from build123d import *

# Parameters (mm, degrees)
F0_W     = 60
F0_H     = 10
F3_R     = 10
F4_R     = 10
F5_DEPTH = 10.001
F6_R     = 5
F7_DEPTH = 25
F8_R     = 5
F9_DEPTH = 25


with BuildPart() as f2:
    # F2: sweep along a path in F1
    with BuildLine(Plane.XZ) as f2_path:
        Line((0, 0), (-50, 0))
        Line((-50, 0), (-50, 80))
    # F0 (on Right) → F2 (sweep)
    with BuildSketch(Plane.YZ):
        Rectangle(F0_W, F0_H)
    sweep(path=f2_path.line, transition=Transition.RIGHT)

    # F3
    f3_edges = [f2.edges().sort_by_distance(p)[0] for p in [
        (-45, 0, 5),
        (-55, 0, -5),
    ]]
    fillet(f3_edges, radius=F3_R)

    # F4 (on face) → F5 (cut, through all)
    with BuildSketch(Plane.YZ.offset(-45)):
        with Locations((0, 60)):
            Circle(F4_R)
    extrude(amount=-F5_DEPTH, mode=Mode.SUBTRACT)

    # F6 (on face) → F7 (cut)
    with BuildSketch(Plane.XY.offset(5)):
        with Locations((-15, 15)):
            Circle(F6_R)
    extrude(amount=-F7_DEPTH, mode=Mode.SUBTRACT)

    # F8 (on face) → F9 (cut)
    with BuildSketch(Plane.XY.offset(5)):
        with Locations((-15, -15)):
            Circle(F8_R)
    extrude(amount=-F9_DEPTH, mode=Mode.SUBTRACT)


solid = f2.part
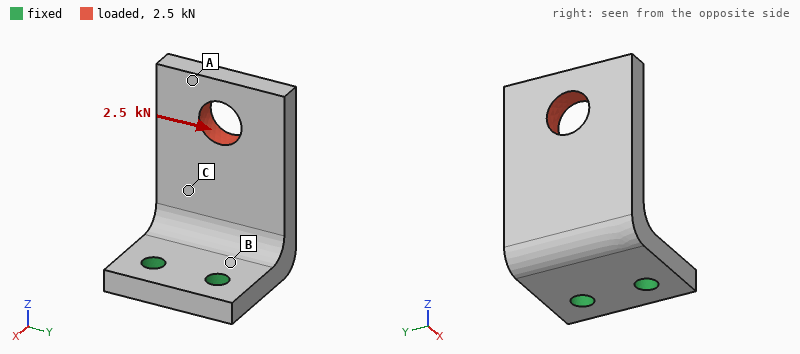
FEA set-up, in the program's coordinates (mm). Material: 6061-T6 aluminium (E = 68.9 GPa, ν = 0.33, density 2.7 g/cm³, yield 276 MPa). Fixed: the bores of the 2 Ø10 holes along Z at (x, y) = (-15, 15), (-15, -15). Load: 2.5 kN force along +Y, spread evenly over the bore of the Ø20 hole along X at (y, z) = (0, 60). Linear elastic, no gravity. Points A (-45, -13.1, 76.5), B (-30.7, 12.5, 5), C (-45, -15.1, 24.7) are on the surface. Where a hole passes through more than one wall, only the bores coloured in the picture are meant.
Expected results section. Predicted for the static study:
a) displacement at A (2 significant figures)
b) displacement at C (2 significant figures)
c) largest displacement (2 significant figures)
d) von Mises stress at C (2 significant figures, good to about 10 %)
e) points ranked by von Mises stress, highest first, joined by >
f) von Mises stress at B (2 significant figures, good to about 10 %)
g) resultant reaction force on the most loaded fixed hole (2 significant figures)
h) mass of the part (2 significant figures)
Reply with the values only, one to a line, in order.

0.35 mm
0.13 mm
0.39 mm
27 MPa
B > C > A
70 MPa
4.4 kN
200 g
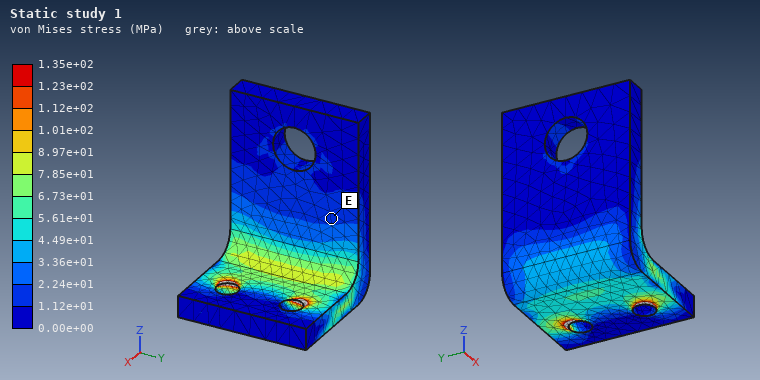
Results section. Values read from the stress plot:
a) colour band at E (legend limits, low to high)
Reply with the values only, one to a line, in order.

1.12e+01 to 2.24e+01 MPa
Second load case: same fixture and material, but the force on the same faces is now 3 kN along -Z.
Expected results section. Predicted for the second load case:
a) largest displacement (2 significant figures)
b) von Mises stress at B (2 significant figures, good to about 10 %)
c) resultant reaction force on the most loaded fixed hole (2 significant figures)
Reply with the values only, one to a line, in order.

0.38 mm
54 MPa
1.5 kN
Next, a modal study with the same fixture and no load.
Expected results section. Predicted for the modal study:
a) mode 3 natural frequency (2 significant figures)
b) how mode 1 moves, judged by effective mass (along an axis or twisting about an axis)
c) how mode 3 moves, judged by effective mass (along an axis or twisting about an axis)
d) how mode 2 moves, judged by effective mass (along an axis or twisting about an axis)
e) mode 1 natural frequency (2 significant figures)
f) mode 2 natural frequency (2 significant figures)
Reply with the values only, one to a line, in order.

3300 Hz
along X
along Z
along Y
920 Hz
1700 Hz
